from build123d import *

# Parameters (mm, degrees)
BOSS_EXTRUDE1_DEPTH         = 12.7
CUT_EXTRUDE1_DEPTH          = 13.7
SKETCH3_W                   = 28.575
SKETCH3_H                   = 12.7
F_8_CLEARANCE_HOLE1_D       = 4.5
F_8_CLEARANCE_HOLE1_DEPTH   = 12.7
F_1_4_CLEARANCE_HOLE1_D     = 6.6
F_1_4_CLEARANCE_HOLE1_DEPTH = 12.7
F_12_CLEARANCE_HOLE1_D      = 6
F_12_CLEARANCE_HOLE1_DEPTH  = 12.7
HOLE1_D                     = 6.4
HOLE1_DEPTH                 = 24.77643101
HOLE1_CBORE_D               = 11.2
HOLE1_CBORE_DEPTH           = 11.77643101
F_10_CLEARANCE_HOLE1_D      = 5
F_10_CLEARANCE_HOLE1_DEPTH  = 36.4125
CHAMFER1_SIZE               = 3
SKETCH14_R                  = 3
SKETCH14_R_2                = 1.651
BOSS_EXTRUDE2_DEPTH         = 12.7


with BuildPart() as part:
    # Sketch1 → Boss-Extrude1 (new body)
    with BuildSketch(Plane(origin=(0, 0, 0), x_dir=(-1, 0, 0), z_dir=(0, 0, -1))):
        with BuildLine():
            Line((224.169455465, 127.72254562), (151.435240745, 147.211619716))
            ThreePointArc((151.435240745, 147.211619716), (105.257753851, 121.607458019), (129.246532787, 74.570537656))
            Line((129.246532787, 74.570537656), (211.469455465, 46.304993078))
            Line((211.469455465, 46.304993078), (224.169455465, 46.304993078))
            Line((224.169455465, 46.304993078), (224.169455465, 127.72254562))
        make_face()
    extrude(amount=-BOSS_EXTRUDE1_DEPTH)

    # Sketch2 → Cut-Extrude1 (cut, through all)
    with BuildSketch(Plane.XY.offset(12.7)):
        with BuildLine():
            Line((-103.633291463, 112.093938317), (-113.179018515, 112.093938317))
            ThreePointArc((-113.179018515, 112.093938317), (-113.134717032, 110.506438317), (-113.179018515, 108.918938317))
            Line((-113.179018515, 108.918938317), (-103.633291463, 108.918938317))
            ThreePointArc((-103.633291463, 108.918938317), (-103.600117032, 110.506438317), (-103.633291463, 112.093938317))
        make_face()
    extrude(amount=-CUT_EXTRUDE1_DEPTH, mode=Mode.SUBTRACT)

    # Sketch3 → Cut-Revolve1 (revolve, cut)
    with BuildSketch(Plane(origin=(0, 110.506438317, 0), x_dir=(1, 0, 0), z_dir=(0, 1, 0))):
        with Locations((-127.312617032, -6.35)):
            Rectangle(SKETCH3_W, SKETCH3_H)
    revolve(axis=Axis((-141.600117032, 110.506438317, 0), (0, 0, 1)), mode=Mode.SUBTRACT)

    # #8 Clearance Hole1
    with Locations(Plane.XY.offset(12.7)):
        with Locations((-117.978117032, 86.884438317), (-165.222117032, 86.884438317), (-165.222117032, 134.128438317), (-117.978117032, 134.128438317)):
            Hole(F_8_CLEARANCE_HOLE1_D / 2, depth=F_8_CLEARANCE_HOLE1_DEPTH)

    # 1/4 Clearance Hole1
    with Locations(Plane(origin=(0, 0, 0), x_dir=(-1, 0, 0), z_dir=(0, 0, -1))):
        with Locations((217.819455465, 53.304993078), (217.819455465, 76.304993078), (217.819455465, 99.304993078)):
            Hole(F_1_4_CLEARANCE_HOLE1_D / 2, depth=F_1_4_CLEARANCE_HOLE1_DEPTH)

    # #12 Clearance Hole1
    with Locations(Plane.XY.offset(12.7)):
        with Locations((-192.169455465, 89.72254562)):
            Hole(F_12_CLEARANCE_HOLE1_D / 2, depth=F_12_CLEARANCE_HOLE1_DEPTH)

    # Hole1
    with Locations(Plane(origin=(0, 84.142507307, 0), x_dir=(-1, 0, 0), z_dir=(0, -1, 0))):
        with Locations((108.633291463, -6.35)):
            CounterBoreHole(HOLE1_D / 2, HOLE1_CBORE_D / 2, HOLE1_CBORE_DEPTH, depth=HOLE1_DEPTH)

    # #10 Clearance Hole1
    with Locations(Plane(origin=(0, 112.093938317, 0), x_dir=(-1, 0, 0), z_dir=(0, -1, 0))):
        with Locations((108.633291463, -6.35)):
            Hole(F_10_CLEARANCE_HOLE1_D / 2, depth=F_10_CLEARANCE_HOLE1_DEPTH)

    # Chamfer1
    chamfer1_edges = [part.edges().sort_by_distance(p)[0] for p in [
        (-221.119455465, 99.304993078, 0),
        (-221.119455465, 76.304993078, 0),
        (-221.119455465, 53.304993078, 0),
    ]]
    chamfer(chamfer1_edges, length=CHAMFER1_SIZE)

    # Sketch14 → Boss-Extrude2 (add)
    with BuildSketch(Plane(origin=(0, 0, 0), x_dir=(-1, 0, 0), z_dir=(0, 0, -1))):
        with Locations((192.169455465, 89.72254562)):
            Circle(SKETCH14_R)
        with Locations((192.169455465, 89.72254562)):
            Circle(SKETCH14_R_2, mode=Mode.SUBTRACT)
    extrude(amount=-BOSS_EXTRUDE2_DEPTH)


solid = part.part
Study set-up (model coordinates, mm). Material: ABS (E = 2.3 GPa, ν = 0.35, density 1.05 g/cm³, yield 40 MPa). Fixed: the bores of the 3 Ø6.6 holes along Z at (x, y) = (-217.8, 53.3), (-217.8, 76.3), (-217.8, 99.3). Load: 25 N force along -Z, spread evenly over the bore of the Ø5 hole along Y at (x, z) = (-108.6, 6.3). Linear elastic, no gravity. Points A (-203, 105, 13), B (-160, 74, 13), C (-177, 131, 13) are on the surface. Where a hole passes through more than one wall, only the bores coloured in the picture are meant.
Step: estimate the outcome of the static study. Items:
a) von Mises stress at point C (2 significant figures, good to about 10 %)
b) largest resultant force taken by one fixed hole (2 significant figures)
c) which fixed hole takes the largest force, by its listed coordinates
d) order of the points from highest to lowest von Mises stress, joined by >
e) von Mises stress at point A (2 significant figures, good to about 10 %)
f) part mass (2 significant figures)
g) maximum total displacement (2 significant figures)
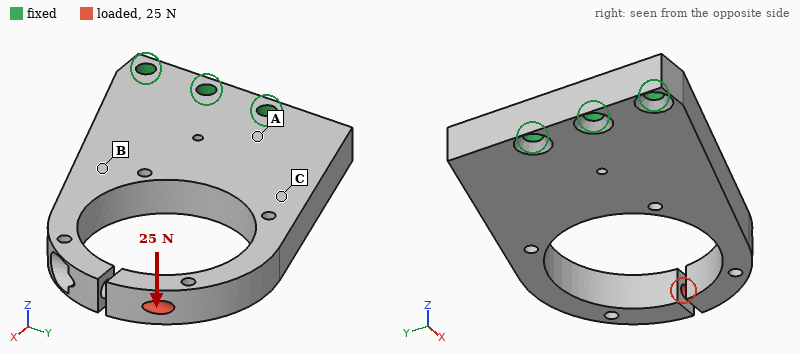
2.8 MPa
26 N
(-217.8, 99.3)
C > A > B
1.5 MPa
82 g
1.9 mm
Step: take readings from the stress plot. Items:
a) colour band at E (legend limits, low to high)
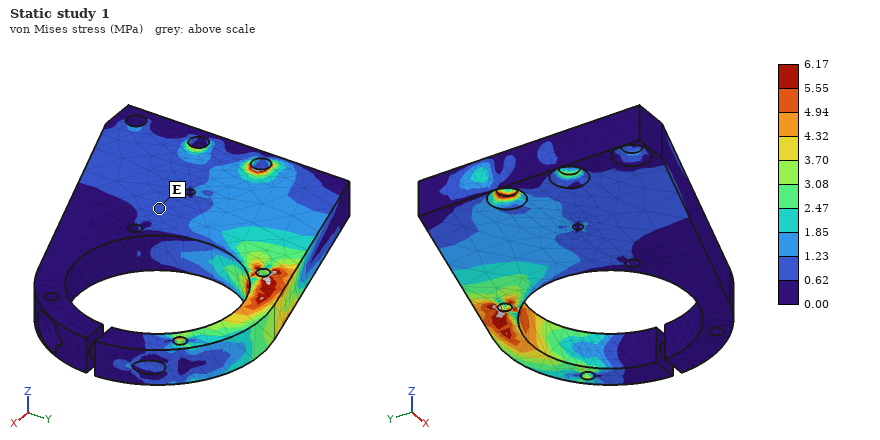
0.62 to 1.23 MPa
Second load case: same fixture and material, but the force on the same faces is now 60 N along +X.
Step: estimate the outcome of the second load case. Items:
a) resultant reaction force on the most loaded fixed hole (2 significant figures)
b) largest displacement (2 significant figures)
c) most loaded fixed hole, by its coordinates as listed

82 N
1.5 mm
(-217.8, 99.3)
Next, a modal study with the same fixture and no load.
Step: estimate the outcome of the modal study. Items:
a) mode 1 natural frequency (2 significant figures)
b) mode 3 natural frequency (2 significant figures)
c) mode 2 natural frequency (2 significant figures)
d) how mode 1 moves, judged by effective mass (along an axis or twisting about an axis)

300 Hz
470 Hz
450 Hz
along Z
